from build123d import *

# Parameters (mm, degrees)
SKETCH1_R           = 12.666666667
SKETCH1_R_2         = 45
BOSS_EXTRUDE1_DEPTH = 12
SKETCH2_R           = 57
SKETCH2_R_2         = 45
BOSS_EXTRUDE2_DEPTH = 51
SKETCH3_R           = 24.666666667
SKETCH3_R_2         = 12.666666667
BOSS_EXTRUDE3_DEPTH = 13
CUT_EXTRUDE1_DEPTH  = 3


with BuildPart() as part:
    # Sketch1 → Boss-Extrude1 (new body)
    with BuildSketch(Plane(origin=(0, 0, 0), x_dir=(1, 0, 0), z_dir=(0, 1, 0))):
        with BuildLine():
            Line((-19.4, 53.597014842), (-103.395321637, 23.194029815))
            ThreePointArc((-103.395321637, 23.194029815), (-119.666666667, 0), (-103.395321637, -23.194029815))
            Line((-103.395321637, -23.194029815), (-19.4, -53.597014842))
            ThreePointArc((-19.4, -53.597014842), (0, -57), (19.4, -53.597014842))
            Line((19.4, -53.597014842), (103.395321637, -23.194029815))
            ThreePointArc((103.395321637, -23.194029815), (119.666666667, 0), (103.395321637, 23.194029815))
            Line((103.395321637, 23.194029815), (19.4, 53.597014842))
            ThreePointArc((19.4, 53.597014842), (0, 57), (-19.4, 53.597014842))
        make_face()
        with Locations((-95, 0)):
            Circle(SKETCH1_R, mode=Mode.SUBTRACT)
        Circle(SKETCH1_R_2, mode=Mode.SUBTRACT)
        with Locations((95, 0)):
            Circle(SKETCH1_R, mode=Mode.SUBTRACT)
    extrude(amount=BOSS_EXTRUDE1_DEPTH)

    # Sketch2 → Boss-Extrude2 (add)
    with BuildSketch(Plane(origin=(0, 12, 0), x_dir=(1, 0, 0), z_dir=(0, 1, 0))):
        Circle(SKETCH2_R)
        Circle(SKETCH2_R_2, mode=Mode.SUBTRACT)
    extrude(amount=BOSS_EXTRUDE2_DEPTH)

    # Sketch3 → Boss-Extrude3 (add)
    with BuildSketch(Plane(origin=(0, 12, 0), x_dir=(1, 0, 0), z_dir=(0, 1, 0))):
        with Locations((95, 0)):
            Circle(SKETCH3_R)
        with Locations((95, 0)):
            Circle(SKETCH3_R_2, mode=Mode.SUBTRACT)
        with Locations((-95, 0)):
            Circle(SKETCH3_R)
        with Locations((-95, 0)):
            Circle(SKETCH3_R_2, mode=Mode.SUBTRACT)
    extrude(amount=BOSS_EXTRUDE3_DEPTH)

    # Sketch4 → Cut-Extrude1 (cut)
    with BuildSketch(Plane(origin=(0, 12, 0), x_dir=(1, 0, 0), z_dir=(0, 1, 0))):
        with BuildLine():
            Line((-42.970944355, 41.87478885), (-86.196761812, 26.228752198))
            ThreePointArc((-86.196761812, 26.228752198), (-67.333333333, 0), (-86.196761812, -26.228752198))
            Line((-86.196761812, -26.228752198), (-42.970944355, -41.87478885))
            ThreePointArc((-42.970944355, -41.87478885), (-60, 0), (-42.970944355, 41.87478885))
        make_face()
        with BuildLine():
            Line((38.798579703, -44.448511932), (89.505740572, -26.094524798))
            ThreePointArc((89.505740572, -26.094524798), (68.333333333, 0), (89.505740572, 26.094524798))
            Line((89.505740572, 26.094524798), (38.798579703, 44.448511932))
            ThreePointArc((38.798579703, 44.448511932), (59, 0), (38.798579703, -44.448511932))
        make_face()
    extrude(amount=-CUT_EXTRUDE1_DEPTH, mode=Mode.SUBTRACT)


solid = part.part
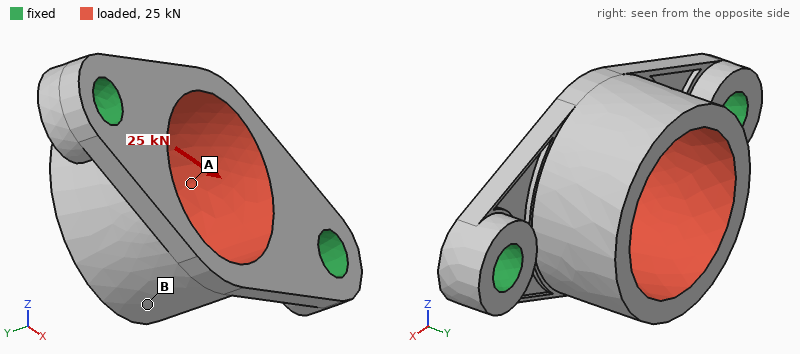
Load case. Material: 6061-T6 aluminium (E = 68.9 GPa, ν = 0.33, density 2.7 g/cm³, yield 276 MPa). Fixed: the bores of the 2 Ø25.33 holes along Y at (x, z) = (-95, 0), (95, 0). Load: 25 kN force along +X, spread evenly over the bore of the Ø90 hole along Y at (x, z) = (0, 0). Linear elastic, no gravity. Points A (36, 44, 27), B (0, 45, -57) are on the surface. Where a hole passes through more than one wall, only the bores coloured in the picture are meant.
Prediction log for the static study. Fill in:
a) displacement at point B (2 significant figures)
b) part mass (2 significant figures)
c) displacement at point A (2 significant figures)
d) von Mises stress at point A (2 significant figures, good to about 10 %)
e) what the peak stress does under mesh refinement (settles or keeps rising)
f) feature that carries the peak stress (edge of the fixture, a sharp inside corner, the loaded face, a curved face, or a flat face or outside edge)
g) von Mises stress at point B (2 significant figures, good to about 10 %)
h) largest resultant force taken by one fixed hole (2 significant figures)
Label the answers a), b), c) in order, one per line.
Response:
a) 48 µm
b) 960 g
c) 53 µm
d) 10 MPa
e) keeps rising
f) edge of the fixture
g) 6.0 MPa
h) 14 kN
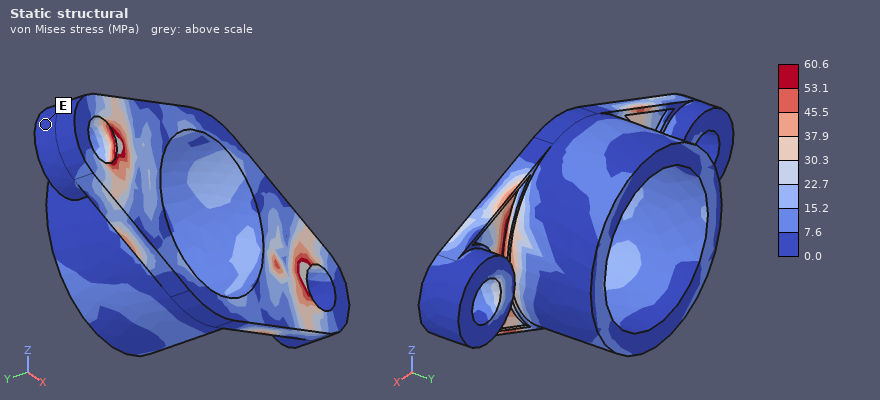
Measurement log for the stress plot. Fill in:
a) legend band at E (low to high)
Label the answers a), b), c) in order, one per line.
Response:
a) 0.0 to 7.6 MPa
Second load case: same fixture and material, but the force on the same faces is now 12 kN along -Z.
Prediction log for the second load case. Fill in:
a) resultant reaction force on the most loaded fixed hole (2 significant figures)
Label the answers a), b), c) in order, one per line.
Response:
a) 6.0 kN
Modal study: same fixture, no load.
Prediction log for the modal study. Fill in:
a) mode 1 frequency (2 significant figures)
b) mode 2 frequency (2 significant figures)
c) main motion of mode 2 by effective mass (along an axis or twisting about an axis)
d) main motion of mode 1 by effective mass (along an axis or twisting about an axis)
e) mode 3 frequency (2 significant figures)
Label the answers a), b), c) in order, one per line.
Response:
a) 1100 Hz
b) 2200 Hz
c) along Y
d) along Z
e) 3700 Hz
